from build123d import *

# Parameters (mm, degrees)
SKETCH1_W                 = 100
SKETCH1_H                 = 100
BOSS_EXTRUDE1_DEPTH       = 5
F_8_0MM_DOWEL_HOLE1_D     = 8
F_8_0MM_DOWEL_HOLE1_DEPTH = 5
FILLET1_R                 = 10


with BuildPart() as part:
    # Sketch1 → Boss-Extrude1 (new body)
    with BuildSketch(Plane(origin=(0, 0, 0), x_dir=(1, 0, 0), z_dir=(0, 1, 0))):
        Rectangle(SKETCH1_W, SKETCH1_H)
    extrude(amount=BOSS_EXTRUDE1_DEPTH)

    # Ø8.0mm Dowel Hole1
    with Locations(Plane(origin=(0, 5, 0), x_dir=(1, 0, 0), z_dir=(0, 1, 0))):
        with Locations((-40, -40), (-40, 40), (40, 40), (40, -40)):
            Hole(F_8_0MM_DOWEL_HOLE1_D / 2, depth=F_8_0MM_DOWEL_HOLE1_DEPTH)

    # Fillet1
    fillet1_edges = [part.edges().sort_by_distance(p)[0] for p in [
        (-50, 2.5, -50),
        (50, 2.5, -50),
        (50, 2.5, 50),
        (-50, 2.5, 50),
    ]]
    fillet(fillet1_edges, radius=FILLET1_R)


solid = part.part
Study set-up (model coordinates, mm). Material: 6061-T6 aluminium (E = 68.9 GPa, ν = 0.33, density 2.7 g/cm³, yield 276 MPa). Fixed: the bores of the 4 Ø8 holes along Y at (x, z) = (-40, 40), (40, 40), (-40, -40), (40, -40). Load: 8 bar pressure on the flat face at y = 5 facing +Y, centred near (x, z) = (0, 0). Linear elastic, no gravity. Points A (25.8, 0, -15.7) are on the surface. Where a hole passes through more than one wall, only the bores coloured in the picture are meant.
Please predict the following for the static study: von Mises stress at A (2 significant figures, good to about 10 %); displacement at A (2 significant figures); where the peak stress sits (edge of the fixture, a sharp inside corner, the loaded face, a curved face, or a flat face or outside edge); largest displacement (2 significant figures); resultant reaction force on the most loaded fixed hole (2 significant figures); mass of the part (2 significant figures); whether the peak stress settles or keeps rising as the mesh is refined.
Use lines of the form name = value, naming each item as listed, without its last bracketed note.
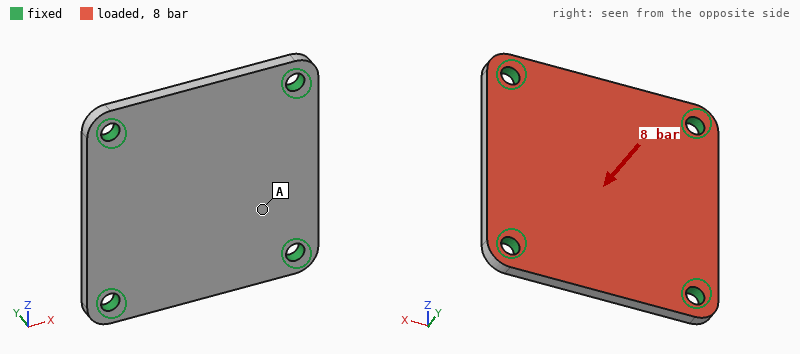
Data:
von Mises stress at A = 35 MPa
displacement at A = 0.16 mm
where the peak stress sits = edge of the fixture
largest displacement = 0.26 mm
resultant reaction force on the most loaded fixed hole = 1.9 kN
mass of the part = 130 g
whether the peak stress settles or keeps rising as the mesh is refined = keeps rising
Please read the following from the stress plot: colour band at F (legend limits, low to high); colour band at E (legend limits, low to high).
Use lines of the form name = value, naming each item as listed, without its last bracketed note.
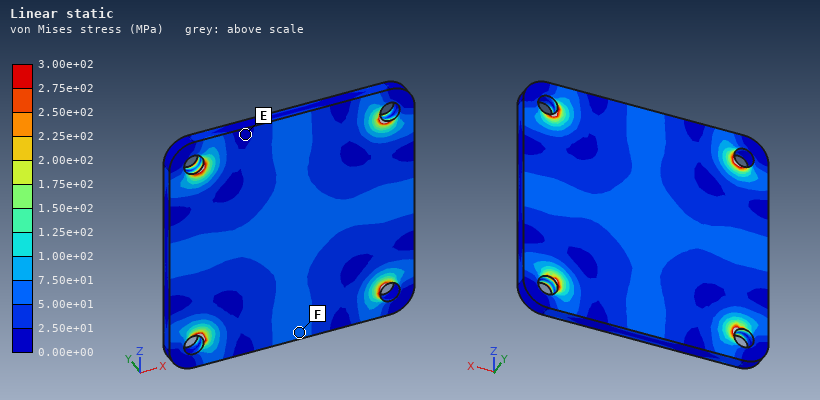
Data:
colour band at F = 5.00e+01 to 7.50e+01 MPa
colour band at E = 0.00e+00 to 2.50e+01 MPa
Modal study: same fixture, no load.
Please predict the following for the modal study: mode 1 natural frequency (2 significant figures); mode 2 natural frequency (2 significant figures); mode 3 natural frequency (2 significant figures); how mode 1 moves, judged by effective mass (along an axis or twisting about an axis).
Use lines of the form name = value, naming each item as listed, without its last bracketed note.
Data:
mode 1 natural frequency = 3000 Hz
mode 2 natural frequency = 4800 Hz
mode 3 natural frequency = 4800 Hz
how mode 1 moves, judged by effective mass = along Y
